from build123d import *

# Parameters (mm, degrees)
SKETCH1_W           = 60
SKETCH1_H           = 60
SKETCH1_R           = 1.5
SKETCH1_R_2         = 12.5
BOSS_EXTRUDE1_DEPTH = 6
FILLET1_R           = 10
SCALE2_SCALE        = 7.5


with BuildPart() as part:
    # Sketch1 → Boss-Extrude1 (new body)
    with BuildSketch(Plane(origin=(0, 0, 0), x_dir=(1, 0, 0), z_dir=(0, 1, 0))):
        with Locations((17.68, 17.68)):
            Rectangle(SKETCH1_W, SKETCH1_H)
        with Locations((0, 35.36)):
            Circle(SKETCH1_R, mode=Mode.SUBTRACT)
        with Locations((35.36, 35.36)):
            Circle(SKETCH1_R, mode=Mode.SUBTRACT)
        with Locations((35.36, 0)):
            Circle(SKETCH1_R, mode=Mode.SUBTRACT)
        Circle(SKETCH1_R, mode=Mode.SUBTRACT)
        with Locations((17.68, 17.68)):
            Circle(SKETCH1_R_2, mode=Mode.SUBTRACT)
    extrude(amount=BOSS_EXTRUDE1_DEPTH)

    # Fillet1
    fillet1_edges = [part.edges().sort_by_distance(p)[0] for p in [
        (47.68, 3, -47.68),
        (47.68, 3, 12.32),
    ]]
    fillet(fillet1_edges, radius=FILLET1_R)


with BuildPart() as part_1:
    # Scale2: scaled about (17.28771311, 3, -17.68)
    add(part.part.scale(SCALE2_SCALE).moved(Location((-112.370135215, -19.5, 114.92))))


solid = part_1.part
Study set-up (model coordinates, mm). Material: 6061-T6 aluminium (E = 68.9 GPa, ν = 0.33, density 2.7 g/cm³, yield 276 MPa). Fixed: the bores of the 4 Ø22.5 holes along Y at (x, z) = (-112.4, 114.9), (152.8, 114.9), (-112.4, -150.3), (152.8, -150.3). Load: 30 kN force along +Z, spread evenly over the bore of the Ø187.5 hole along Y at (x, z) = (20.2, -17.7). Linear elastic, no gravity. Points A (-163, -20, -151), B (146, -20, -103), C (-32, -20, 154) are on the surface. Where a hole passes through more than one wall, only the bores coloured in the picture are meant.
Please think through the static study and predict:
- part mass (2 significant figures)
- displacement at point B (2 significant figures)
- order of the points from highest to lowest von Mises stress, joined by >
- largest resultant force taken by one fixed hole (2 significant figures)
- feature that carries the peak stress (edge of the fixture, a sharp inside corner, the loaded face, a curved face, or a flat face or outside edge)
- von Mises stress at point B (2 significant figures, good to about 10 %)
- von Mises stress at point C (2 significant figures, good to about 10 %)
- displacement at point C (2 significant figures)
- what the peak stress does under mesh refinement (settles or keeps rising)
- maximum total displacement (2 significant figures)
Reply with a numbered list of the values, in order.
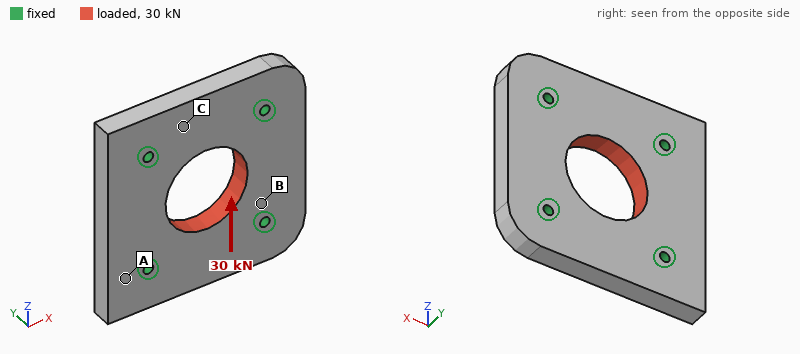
1. 21 kg
2. 1.1 µm
3. B > C > A
4. 7.6 kN
5. edge of the fixture
6. 1.6 MPa
7. 0.97 MPa
8. 3.0 µm
9. keeps rising
10. 4.6 µm
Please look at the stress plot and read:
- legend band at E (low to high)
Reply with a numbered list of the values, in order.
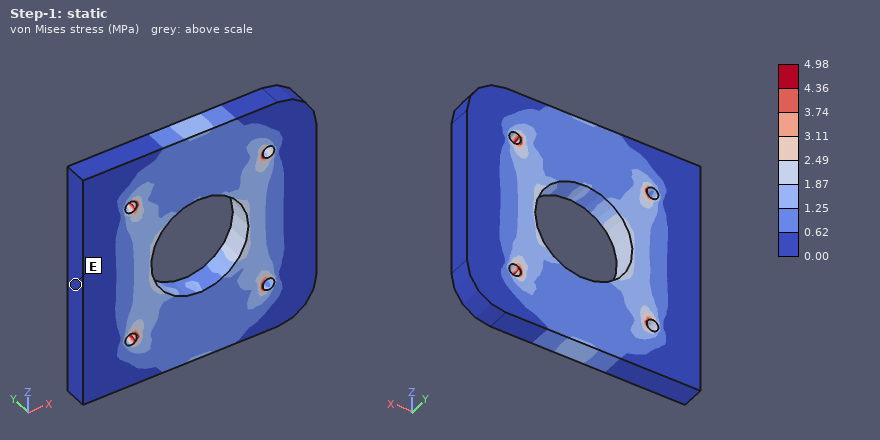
1. 0.00 to 0.62 MPa
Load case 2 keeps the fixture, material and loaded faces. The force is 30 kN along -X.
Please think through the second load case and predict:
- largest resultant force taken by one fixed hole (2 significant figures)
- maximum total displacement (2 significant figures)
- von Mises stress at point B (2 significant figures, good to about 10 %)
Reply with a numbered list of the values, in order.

1. 7.6 kN
2. 4.6 µm
3. 1.2 MPa
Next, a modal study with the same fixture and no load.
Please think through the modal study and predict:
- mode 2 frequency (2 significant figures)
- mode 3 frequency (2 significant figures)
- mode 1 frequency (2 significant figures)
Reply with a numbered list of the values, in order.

1. 2200 Hz
2. 2200 Hz
3. 1900 Hz
